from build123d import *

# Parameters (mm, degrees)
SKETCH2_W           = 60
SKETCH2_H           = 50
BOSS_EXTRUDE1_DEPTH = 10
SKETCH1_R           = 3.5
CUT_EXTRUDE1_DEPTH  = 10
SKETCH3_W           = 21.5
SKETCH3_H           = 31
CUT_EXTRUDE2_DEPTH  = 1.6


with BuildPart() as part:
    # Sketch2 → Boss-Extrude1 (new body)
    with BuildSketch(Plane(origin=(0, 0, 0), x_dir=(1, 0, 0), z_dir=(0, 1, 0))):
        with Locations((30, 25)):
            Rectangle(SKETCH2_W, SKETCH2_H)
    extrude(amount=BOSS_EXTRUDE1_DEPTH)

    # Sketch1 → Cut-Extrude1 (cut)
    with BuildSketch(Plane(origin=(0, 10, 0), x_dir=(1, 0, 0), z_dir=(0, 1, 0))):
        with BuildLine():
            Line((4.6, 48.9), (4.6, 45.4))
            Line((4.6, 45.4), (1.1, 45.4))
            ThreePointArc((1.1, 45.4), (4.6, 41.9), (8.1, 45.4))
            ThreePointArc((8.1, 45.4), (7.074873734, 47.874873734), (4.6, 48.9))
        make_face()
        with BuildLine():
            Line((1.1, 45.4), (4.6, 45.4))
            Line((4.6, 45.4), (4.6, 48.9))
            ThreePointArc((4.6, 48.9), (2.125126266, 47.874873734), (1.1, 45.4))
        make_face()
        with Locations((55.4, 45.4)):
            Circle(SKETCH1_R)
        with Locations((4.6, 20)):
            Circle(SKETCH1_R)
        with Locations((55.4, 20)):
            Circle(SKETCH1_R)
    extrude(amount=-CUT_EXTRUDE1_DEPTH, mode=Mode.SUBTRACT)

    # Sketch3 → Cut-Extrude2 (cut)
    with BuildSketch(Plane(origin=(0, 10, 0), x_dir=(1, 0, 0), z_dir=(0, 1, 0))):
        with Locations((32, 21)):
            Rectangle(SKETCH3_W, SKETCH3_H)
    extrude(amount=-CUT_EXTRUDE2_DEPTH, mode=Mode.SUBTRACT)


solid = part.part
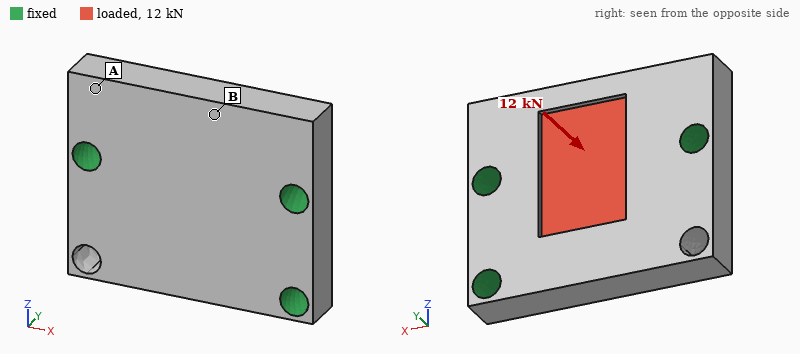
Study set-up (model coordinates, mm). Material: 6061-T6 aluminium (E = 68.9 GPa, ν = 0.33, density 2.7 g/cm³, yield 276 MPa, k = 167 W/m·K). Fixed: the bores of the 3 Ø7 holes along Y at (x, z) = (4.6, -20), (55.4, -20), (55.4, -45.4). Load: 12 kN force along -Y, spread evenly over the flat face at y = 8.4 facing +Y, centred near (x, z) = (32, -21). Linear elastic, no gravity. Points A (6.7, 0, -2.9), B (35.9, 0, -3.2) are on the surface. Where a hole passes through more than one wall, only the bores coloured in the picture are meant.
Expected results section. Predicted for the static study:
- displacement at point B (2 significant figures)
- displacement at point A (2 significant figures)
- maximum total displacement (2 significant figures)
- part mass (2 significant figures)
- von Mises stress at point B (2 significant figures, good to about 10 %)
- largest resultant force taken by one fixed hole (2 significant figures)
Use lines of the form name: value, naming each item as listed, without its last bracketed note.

displacement at point B: 59 µm
displacement at point A: 18 µm
maximum total displacement: 66 µm
part mass: 74 g
von Mises stress at point B: 69 MPa
largest resultant force taken by one fixed hole: 5.6 kN
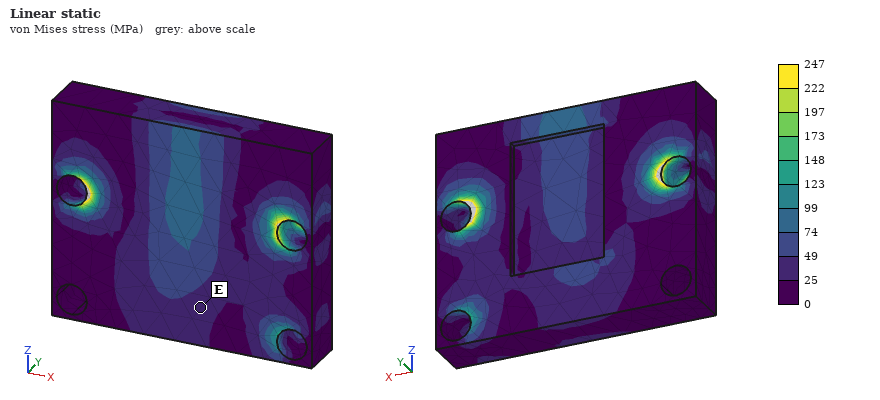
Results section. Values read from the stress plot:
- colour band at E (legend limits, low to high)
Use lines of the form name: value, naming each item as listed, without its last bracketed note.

colour band at E: 25 to 49 MPa
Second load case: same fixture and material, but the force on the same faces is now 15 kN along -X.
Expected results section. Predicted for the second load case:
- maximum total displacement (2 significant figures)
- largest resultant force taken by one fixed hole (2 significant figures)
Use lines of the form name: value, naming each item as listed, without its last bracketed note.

maximum total displacement: 14 µm
largest resultant force taken by one fixed hole: 6.5 kN
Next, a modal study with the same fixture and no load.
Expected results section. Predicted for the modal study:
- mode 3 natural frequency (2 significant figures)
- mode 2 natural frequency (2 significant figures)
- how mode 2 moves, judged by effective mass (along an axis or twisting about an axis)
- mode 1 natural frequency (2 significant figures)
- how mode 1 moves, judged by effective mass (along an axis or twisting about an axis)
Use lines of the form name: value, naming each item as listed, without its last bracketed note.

mode 3 natural frequency: 20 kHz
mode 2 natural frequency: 13 kHz
how mode 2 moves, judged by effective mass: along Y
mode 1 natural frequency: 10 kHz
how mode 1 moves, judged by effective mass: along Y
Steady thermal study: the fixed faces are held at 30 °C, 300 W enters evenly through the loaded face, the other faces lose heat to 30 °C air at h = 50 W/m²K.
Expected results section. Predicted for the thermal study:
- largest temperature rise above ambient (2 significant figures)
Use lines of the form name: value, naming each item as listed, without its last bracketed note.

largest temperature rise above ambient: 59 K
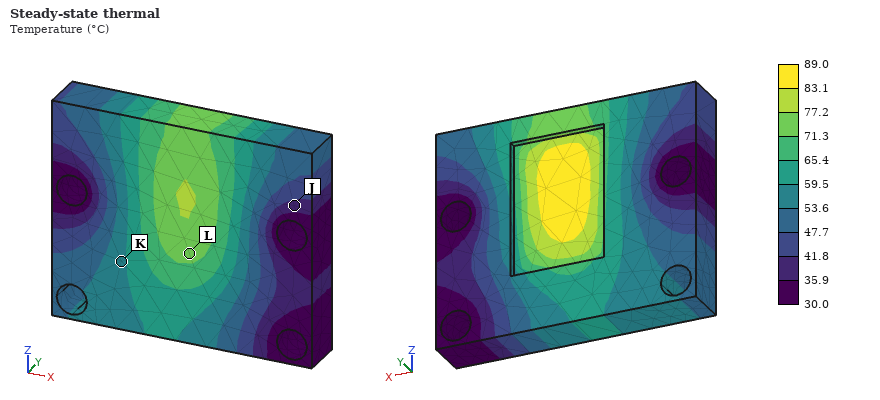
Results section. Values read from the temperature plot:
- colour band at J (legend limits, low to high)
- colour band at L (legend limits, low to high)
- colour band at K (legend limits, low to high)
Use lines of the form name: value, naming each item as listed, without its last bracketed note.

colour band at J: 35.9 to 41.8 °C
colour band at L: 71.3 to 77.2 °C
colour band at K: 53.6 to 59.5 °C
